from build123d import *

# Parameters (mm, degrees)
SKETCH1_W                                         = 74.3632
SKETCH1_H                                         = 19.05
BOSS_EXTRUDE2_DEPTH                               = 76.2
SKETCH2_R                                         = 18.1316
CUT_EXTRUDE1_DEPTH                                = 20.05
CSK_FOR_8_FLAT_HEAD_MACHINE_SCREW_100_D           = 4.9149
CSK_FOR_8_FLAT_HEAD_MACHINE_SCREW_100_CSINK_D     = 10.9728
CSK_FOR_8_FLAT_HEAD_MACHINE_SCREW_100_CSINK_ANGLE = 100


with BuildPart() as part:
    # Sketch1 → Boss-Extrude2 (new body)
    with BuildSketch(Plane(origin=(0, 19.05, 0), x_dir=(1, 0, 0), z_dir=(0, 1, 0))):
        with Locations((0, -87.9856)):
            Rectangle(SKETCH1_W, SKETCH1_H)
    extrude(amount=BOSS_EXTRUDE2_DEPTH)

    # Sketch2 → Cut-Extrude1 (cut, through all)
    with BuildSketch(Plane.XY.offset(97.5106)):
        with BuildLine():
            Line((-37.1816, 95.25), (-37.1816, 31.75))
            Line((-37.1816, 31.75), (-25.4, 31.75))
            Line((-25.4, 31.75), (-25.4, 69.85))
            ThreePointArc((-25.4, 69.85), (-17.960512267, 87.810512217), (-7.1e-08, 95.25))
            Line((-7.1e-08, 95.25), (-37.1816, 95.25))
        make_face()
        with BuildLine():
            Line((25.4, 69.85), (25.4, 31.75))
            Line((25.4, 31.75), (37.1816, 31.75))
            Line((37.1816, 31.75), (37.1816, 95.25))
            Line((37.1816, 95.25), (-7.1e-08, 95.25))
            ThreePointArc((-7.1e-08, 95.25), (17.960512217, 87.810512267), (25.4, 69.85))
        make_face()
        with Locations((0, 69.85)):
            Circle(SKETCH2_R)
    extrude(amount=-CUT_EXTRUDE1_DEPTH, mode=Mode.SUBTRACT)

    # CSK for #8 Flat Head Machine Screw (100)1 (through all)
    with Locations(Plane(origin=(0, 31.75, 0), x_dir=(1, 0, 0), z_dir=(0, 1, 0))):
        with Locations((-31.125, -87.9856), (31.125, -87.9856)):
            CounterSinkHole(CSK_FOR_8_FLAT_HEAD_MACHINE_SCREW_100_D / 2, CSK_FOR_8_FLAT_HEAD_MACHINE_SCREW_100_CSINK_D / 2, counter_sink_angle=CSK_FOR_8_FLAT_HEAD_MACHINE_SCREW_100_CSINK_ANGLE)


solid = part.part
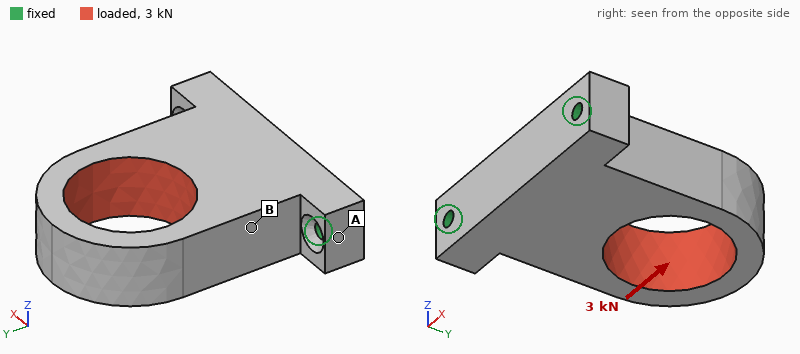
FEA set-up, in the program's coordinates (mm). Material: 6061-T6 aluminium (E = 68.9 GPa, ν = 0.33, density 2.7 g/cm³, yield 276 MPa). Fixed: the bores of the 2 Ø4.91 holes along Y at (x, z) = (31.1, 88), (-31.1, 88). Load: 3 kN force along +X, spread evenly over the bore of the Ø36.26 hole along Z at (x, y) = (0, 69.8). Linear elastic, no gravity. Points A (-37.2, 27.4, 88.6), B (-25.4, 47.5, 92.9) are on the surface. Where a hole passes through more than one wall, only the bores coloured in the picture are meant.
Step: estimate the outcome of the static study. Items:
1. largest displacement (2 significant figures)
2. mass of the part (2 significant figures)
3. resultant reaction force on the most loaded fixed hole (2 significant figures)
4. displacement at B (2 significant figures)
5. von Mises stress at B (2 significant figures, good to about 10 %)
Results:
73 µm
150 g
2.8 kN
13 µm
23 MPa
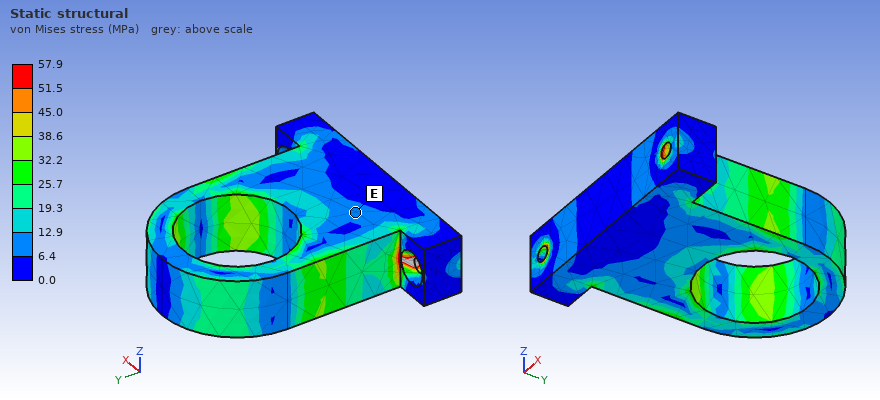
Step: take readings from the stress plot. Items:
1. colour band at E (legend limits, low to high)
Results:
6.4 to 12.9 MPa
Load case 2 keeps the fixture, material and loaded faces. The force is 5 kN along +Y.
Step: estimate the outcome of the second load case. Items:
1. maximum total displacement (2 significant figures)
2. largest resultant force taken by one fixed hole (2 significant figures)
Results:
25 µm
2.7 kN
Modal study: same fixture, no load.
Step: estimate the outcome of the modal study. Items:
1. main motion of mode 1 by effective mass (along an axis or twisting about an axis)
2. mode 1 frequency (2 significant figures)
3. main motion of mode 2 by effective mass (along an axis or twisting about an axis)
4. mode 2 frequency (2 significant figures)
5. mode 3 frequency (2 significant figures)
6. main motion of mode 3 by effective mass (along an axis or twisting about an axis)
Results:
along Z
2100 Hz
along X
5000 Hz
7100 Hz
twisting about Y
